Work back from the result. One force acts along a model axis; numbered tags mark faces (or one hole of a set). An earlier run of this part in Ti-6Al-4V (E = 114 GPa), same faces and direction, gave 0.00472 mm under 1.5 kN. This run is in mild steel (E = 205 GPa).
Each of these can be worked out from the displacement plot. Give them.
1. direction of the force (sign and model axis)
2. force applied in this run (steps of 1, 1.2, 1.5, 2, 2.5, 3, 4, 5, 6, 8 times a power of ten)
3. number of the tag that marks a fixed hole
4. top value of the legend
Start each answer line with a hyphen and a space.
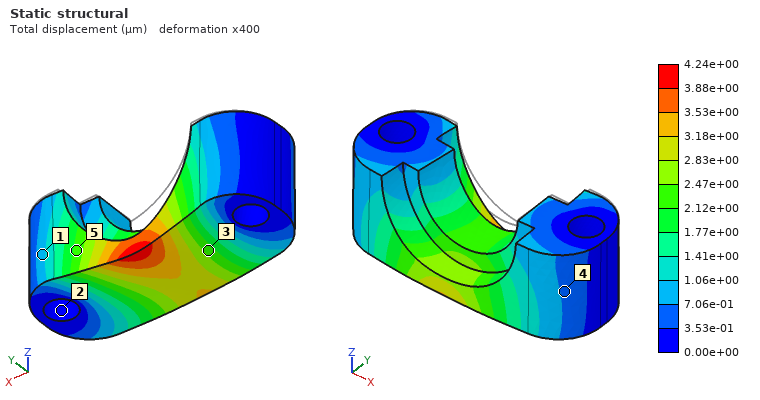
- -Y
- 2.5 kN
- 2
- 4.24e+00 µm
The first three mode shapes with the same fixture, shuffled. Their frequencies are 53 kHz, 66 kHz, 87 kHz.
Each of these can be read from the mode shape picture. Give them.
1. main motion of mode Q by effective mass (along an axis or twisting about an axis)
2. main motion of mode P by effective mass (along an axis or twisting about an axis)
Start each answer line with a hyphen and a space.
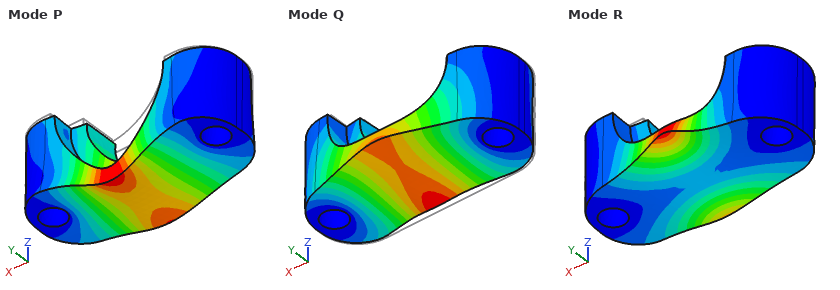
- along Y
- along Z
